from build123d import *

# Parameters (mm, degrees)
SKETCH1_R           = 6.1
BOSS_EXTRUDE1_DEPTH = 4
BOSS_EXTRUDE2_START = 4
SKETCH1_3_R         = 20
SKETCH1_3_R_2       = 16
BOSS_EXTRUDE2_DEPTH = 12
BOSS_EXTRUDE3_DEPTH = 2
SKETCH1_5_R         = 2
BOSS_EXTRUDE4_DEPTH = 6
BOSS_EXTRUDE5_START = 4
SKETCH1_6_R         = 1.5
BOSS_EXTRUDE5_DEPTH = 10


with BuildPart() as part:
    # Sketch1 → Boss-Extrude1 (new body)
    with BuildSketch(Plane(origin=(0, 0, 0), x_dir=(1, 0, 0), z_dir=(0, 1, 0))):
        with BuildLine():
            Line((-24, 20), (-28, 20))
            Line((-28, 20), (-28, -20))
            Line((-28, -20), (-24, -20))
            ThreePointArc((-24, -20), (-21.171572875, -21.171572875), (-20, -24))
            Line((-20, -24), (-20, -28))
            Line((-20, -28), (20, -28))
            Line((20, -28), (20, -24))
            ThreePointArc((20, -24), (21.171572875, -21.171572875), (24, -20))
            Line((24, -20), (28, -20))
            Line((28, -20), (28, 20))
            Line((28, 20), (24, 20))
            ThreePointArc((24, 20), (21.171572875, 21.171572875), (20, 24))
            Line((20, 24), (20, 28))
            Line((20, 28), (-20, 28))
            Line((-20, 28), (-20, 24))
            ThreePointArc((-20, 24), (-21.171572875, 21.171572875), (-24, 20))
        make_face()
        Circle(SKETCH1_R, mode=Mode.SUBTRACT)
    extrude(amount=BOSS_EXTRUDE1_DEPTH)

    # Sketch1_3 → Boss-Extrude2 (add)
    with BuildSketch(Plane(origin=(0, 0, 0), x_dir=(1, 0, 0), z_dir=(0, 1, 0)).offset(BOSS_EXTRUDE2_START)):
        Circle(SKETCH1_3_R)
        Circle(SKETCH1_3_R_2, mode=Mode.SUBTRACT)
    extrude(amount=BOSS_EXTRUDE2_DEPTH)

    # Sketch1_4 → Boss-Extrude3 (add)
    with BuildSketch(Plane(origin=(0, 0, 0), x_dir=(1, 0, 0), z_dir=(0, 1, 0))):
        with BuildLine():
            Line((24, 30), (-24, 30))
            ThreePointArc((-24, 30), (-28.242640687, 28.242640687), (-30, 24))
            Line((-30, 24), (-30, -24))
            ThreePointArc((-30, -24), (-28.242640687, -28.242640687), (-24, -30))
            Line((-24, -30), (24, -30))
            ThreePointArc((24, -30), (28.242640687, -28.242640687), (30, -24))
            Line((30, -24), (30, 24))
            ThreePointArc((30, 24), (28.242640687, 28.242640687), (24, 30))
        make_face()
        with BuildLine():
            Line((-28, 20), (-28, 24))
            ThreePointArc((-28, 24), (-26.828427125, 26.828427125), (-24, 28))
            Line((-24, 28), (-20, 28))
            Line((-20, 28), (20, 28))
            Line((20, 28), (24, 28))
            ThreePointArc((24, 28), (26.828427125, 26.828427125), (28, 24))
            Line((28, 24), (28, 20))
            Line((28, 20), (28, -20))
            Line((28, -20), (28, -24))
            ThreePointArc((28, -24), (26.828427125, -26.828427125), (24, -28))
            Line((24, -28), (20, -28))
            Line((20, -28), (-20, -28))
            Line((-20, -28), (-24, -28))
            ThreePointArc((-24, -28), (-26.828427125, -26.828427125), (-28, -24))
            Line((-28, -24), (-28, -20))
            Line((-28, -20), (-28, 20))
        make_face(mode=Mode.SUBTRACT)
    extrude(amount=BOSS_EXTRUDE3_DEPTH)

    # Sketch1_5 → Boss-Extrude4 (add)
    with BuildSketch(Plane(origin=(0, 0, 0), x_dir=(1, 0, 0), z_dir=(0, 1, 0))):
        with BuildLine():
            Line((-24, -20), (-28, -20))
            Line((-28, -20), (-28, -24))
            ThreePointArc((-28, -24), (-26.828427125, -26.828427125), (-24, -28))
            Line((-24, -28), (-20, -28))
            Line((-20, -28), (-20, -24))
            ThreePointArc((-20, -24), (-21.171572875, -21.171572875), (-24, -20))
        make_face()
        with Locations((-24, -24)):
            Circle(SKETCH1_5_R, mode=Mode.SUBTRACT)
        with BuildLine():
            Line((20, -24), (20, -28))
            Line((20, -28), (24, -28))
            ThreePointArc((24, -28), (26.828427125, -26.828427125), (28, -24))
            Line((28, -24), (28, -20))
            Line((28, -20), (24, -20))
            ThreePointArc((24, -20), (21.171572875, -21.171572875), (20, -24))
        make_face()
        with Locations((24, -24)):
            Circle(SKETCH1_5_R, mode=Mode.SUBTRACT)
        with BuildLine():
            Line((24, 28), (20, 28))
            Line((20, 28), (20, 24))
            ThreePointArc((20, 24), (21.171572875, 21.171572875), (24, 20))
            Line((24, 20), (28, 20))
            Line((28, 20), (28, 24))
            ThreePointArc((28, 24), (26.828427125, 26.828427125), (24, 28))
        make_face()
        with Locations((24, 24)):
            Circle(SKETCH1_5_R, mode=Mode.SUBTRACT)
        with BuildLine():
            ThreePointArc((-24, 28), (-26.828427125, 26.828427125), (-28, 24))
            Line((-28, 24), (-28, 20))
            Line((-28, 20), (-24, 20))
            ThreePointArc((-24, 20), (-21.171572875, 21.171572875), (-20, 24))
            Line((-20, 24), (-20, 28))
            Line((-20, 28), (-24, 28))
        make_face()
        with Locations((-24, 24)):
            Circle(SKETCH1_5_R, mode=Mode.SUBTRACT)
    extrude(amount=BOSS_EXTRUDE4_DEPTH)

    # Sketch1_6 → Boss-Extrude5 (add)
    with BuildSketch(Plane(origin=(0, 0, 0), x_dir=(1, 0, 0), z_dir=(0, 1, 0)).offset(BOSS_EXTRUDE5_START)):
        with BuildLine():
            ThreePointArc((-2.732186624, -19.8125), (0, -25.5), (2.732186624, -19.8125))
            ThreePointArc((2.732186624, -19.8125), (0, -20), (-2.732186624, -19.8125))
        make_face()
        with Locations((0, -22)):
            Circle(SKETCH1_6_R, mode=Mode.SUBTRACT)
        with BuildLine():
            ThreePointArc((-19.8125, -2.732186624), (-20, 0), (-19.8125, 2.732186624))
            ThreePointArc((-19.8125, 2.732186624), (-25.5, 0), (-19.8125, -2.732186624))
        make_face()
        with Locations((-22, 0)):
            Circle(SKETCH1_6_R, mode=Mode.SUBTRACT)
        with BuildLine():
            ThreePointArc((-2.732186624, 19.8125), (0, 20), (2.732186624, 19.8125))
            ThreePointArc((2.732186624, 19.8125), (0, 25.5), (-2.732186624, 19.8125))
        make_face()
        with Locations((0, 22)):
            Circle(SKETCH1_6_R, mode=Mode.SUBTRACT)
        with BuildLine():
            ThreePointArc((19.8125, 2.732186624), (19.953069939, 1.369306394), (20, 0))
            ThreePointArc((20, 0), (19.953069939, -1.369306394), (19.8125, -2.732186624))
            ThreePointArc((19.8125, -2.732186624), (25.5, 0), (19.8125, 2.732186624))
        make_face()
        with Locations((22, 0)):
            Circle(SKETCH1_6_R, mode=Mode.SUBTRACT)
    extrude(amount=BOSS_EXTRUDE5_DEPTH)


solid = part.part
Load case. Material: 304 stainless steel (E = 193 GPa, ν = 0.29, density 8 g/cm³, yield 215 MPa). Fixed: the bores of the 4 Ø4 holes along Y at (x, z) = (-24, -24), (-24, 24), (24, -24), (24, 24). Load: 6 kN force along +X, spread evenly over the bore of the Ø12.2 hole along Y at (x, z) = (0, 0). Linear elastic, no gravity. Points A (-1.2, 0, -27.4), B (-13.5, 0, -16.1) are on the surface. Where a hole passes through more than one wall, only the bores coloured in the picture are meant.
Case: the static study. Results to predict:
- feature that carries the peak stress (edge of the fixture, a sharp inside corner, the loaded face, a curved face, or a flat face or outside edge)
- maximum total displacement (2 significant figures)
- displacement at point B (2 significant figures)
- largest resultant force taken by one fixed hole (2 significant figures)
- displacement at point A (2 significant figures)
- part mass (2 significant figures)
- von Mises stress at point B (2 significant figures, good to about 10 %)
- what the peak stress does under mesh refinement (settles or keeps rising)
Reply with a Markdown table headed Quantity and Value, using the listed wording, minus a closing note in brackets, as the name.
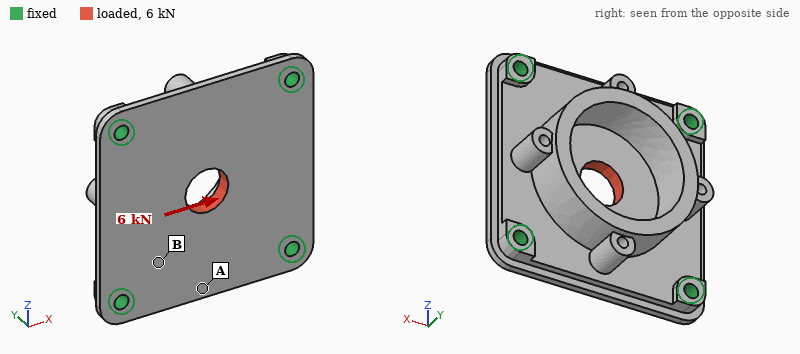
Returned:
| Quantity | Value |
|---|---|
| feature that carries the peak stress | edge of the fixture |
| maximum total displacement | 5.8 µm |
| displacement at point B | 2.4 µm |
| largest resultant force taken by one fixed hole | 1.7 kN |
| displacement at point A | 1.4 µm |
| part mass | 160 g |
| von Mises stress at point B | 26 MPa |
| what the peak stress does under mesh refinement | keeps rising |
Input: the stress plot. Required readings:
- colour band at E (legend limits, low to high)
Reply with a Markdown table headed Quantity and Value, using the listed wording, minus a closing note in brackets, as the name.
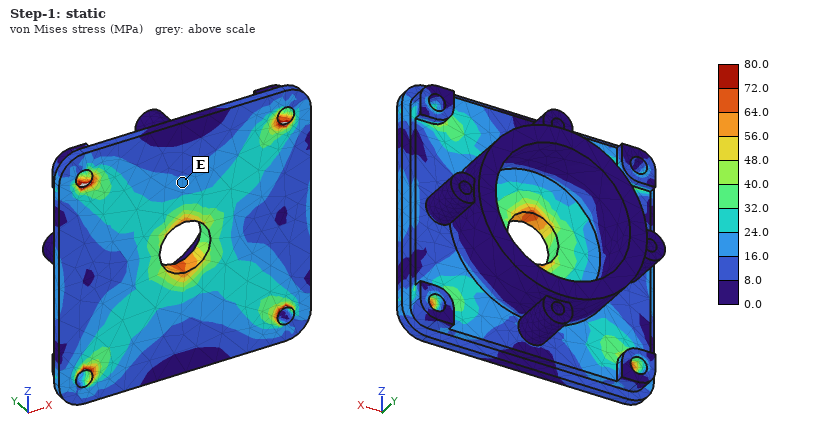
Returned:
| Quantity | Value |
|---|---|
| colour band at E | 16.0 to 24.0 MPa |
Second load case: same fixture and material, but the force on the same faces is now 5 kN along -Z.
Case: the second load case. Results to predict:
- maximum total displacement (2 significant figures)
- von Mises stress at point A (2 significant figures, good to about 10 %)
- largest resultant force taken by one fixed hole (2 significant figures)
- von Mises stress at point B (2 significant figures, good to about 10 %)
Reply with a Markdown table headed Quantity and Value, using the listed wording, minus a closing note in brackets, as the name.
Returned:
| Quantity | Value |
|---|---|
| maximum total displacement | 4.8 µm |
| von Mises stress at point A | 11 MPa |
| largest resultant force taken by one fixed hole | 1.4 kN |
| von Mises stress at point B | 23 MPa |
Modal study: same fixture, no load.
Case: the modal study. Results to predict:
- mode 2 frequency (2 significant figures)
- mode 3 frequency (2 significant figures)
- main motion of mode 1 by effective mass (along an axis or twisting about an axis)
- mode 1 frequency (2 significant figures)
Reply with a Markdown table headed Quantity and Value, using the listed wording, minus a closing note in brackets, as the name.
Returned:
| Quantity | Value |
|---|---|
| mode 2 frequency | 8900 Hz |
| mode 3 frequency | 8900 Hz |
| main motion of mode 1 by effective mass | along Y |
| mode 1 frequency | 6600 Hz |
